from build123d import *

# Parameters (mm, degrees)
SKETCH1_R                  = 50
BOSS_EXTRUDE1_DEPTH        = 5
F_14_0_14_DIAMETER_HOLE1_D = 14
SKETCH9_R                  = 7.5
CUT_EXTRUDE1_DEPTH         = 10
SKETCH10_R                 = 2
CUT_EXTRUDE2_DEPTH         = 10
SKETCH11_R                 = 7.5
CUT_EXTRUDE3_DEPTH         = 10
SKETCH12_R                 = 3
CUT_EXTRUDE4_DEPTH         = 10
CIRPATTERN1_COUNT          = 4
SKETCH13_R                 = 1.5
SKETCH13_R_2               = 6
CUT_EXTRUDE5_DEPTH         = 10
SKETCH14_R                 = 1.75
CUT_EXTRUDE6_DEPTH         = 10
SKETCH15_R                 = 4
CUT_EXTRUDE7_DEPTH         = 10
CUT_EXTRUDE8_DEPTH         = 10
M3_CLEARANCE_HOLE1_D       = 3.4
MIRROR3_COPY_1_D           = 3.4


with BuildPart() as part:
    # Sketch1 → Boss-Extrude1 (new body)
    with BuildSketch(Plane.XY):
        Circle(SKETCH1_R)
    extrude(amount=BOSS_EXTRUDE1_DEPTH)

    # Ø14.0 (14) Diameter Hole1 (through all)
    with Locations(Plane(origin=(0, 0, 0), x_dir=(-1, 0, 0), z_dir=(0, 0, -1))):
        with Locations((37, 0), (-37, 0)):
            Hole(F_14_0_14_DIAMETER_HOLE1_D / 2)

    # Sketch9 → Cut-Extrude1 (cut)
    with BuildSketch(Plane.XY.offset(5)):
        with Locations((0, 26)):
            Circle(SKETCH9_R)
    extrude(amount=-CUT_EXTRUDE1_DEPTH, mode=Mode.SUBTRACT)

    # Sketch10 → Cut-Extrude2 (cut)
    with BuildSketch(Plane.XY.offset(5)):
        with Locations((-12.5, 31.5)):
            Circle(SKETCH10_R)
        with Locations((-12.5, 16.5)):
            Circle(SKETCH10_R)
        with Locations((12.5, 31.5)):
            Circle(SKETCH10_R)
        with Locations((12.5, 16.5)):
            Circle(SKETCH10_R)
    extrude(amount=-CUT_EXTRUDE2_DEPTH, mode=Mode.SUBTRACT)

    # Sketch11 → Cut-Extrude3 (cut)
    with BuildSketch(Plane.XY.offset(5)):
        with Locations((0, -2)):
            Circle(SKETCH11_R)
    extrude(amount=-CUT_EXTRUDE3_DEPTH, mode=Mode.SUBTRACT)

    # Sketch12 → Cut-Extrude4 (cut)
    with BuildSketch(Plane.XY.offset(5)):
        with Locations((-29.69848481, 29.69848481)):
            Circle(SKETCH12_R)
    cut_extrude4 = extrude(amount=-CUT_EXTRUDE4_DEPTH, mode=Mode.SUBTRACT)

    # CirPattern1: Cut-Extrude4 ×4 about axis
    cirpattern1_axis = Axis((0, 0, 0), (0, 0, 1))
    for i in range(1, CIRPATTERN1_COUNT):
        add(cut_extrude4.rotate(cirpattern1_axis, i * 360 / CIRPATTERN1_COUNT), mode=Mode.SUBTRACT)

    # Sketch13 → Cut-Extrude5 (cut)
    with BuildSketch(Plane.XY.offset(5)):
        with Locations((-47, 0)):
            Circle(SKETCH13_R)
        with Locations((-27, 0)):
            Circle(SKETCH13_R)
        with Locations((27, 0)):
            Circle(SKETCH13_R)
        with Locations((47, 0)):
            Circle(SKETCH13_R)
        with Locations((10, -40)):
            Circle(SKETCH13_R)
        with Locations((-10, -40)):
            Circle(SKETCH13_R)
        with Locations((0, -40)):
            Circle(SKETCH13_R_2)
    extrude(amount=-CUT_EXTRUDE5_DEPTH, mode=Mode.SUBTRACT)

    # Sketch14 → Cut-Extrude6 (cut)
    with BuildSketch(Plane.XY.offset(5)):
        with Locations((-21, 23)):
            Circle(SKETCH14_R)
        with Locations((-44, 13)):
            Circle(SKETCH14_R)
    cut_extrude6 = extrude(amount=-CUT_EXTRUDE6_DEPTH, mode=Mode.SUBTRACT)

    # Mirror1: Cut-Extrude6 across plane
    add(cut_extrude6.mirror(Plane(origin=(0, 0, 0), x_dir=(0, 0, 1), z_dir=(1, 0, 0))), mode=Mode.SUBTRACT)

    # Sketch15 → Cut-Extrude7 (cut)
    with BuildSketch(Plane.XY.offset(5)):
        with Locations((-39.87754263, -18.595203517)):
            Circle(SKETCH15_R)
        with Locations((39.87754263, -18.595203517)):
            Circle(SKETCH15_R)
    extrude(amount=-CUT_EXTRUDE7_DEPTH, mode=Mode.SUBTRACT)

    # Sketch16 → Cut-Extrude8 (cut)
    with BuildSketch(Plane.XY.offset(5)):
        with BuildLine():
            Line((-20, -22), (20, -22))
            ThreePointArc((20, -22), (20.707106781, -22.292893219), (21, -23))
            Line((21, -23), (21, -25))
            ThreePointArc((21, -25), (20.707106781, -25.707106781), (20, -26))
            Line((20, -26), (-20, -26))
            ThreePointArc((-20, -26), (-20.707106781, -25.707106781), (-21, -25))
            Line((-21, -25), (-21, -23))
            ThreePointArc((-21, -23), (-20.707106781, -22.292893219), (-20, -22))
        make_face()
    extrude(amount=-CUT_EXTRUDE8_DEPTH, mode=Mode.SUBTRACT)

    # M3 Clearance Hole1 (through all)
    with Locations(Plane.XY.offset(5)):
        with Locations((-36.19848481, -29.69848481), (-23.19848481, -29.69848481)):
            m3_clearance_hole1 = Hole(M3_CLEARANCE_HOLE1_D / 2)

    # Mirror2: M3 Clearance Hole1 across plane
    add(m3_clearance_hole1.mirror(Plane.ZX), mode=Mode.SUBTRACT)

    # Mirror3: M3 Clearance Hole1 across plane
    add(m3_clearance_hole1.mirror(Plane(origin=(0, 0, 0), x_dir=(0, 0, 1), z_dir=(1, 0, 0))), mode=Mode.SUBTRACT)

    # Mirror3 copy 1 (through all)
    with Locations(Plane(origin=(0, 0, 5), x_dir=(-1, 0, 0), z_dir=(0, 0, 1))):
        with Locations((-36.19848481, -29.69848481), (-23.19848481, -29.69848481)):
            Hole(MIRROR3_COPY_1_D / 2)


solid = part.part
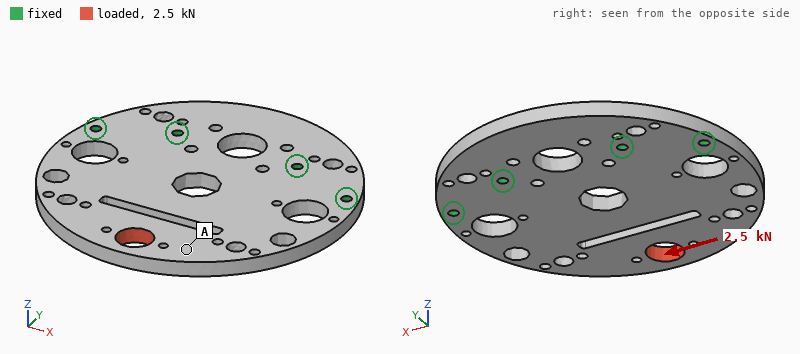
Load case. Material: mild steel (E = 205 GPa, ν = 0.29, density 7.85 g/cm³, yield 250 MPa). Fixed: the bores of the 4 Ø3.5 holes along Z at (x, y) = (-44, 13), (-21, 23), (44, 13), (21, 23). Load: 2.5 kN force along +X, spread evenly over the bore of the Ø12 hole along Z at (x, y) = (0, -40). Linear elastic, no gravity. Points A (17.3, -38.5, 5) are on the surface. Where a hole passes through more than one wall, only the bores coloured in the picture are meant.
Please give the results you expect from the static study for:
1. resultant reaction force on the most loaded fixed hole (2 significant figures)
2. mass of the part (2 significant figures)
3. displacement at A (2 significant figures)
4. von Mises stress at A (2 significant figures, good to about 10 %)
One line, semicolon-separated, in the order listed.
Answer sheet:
1.5 kN; 250 g; 15 µm; 11 MPa
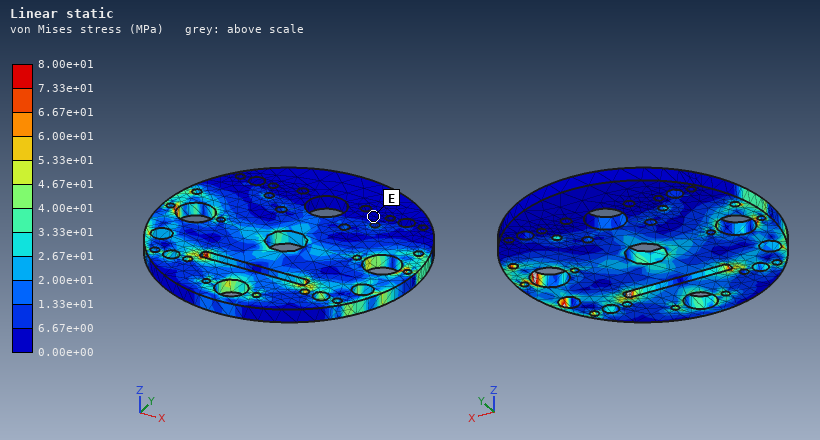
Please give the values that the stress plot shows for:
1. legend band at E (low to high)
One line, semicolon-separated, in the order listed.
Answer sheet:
0.00e+00 to 6.67e+00 MPa
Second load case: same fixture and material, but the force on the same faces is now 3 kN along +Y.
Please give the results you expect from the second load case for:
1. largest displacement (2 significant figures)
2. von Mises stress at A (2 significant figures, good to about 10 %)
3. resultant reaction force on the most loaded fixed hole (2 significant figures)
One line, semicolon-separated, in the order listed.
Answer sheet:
15 µm; 31 MPa; 910 N
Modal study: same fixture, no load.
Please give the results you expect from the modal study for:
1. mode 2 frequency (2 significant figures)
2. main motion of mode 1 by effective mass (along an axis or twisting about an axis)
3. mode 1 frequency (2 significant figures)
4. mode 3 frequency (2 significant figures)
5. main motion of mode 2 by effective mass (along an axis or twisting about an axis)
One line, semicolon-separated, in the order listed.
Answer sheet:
2500 Hz; along Z; 940 Hz; 4100 Hz; twisting about Y
